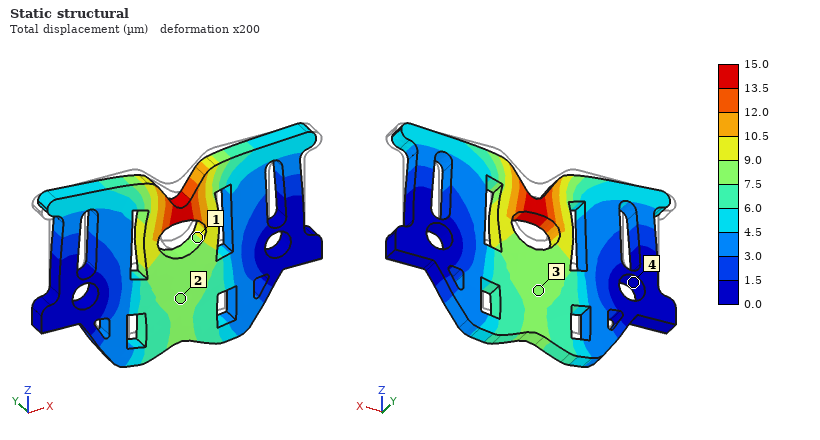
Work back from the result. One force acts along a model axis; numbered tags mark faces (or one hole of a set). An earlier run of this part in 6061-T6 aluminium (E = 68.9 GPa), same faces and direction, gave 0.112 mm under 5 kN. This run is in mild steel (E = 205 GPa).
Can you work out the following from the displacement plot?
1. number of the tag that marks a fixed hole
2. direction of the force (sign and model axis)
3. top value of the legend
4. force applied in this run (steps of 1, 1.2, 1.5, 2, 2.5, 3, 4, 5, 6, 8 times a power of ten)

4
-Z
15.0 µm
2 kN
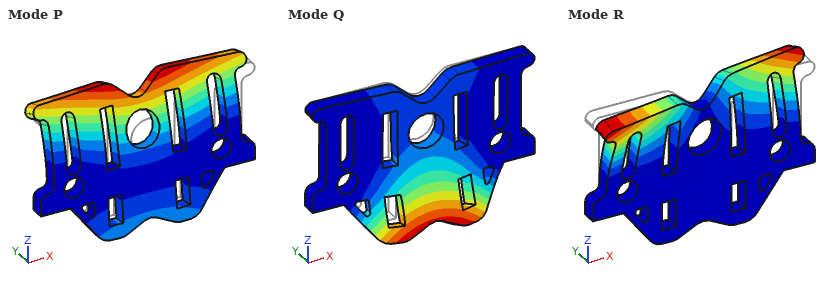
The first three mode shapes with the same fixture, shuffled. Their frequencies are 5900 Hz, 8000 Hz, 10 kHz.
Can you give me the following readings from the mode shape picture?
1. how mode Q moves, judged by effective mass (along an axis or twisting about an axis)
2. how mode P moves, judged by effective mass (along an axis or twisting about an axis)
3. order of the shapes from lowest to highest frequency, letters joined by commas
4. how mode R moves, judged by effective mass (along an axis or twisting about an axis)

along Y
along Y
P, R, Q
twisting about Z
